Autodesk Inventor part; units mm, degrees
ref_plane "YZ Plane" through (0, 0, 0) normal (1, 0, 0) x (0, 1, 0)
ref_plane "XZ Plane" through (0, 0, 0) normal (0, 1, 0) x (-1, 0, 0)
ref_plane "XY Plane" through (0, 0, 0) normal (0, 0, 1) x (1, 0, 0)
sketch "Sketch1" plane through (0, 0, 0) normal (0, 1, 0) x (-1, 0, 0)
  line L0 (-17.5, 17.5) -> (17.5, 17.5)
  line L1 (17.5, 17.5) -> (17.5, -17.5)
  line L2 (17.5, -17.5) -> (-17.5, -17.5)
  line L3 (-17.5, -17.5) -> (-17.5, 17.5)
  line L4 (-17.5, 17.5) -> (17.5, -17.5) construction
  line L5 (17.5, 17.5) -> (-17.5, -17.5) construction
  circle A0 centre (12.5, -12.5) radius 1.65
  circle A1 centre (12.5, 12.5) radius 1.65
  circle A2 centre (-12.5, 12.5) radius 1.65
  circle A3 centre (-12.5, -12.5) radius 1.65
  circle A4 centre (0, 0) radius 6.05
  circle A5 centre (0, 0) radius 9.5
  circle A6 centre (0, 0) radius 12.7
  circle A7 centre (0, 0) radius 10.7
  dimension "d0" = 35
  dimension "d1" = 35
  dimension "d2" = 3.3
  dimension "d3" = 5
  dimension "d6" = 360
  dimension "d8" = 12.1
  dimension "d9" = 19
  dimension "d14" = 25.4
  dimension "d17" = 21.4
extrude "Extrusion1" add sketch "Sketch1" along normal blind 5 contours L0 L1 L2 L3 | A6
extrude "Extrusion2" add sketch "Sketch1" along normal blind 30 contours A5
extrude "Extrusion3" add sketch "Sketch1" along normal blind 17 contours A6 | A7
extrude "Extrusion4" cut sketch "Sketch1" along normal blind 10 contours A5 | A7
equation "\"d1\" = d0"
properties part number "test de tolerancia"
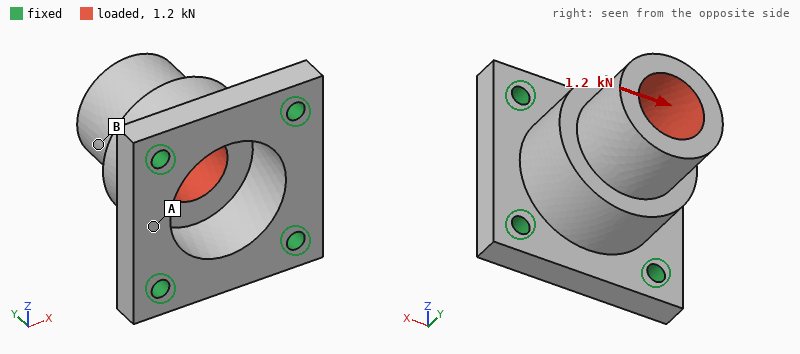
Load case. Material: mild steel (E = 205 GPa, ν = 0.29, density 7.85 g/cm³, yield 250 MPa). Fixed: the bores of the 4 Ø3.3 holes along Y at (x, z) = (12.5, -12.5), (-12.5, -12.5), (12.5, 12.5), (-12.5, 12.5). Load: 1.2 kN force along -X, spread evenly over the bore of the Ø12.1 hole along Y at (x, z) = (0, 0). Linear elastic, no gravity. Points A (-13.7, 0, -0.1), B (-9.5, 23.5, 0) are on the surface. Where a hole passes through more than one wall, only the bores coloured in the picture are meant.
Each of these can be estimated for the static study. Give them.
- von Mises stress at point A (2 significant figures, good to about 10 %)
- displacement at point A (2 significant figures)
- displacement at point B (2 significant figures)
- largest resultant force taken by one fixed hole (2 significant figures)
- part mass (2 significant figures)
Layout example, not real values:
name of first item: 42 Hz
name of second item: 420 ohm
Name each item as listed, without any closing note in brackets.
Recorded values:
von Mises stress at point A: 18 MPa
displacement at point A: 1.9 µm
displacement at point B: 6.3 µm
largest resultant force taken by one fixed hole: 560 N
part mass: 77 g
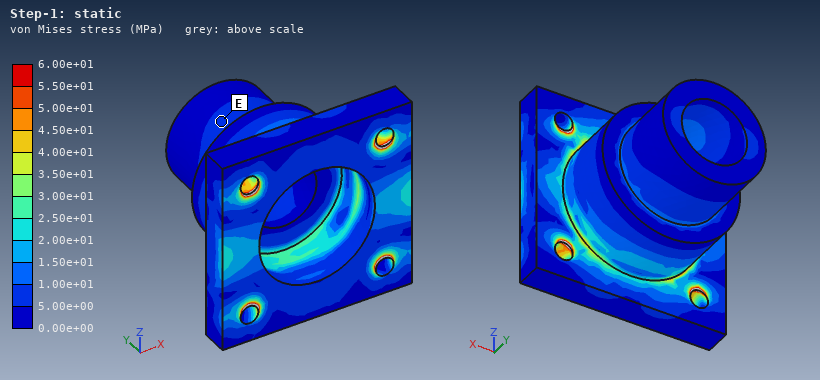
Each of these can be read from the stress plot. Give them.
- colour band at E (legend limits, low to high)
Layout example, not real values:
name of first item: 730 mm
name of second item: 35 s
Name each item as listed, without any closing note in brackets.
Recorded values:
colour band at E: 5.00e+00 to 1.00e+01 MPa
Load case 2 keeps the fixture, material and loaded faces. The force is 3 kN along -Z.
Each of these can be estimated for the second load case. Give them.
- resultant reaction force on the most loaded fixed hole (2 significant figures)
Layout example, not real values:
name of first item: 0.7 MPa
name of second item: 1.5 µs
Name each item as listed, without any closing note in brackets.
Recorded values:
resultant reaction force on the most loaded fixed hole: 1.4 kN
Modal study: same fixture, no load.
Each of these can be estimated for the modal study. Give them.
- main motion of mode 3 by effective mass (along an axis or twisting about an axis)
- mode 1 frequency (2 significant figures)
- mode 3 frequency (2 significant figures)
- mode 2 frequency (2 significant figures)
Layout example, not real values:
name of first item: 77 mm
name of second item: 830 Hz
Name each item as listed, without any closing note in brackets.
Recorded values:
main motion of mode 3 by effective mass: along Y
mode 1 frequency: 13 kHz
mode 3 frequency: 21 kHz
mode 2 frequency: 13 kHz
